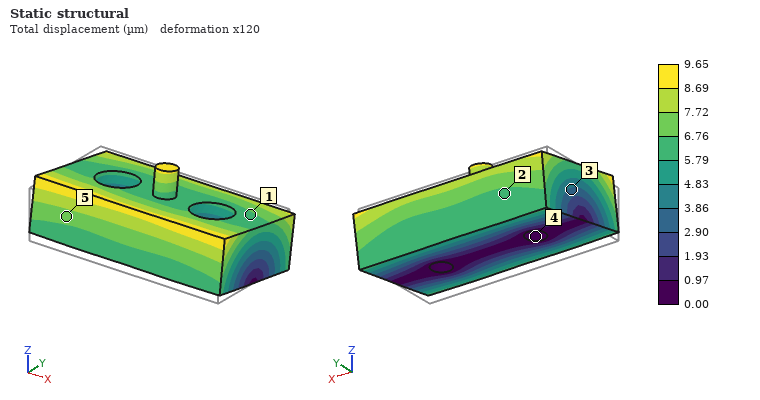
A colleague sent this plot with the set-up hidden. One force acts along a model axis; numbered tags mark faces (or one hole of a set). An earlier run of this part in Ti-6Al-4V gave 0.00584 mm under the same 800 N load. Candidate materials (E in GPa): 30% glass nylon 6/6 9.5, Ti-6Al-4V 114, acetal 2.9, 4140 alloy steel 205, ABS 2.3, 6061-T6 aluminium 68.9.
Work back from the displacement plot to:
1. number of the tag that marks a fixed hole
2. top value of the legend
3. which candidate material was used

4
9.65 µm
6061-T6 aluminium
